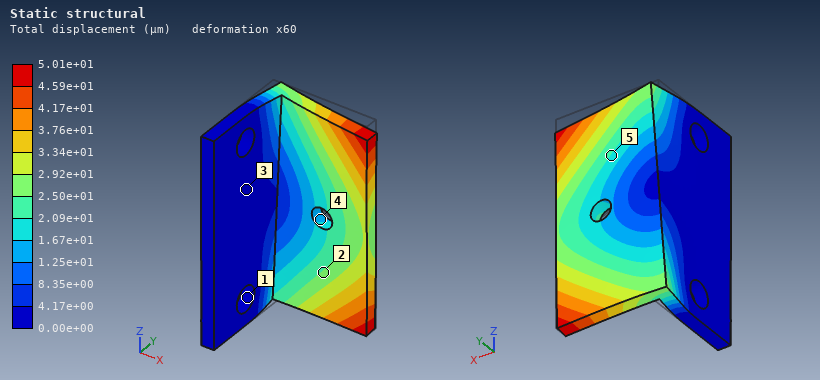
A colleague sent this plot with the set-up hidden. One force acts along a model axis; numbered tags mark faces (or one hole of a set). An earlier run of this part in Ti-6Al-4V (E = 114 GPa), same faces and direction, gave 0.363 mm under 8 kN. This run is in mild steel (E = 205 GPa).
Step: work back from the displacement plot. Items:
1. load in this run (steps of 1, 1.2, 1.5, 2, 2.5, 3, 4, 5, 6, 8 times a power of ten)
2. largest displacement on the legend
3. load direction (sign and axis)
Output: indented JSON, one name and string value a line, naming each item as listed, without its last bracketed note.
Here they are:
{
  "load in this run": "2 kN",
  "largest displacement on the legend": "5.01e+01 µm",
  "load direction": "-Z"
}
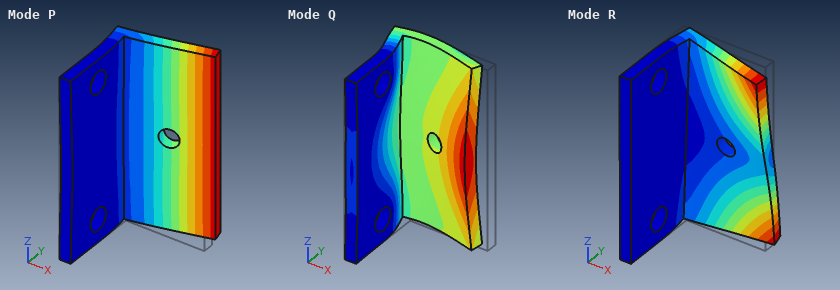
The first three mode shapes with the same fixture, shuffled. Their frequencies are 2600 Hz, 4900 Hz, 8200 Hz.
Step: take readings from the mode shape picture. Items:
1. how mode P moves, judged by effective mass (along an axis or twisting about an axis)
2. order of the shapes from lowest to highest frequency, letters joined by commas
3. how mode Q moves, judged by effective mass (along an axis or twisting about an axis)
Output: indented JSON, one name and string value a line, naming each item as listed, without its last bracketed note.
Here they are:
{
  "how mode P moves, judged by effective mass": "along Y",
  "order of the shapes from lowest to highest frequency, letters joined by commas": "P, R, Q",
  "how mode Q moves, judged by effective mass": "along X"
}
